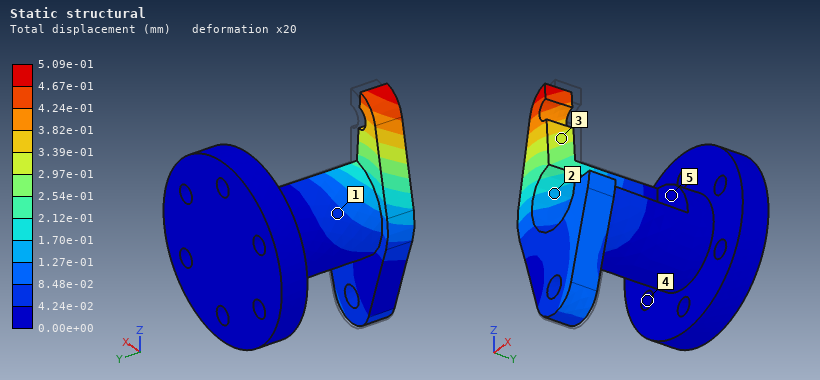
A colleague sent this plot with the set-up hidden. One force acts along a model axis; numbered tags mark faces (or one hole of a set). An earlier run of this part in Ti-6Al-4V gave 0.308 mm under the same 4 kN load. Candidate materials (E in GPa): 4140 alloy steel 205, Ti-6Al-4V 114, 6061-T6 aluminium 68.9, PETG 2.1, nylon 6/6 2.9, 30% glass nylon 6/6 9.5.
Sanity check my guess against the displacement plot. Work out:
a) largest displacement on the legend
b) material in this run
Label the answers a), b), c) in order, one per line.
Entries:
a) 5.09e-01 mm
b) 6061-T6 aluminium
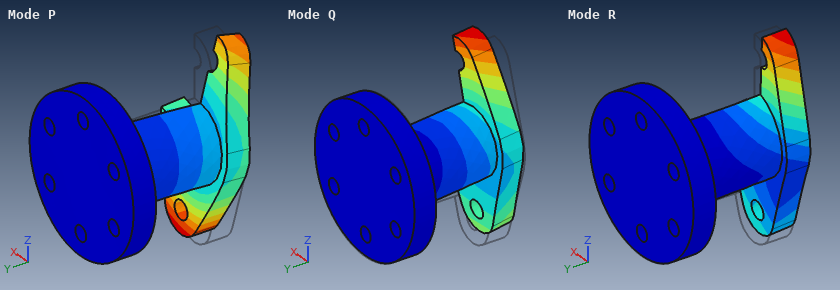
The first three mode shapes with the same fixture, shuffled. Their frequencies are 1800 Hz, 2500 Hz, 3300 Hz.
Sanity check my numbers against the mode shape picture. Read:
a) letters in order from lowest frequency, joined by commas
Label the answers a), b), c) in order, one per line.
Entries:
a) R, Q, P
